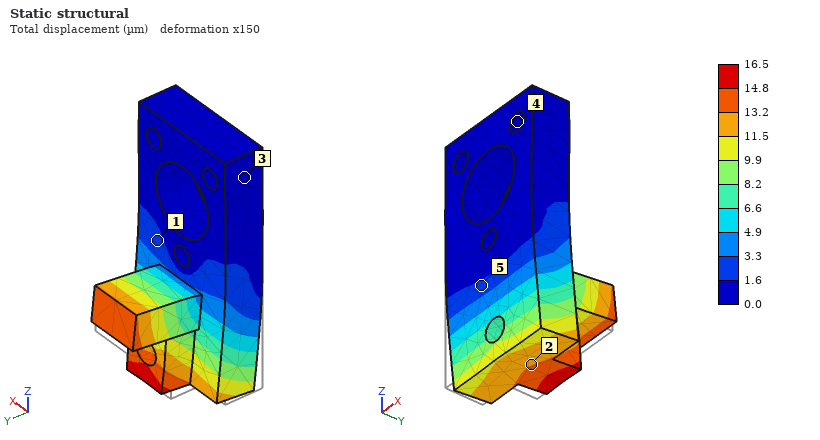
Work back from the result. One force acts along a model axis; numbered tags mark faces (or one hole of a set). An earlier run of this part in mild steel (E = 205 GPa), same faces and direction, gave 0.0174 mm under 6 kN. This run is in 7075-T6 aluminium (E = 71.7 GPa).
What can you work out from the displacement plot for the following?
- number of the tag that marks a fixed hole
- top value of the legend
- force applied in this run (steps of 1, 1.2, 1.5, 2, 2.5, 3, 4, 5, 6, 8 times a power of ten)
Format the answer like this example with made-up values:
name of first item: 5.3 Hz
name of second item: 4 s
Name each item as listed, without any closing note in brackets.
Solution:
number of the tag that marks a fixed hole: 4
top value of the legend: 16.5 µm
force applied in this run: 2 kN
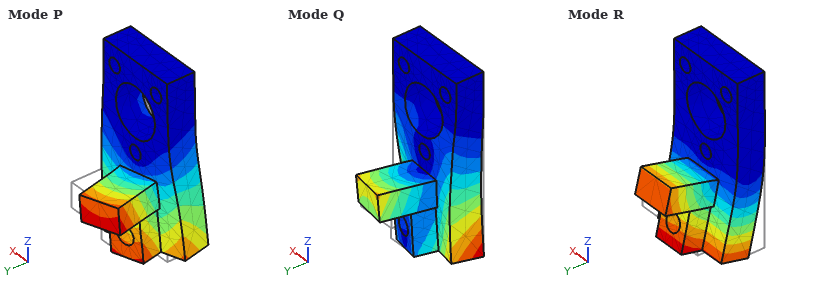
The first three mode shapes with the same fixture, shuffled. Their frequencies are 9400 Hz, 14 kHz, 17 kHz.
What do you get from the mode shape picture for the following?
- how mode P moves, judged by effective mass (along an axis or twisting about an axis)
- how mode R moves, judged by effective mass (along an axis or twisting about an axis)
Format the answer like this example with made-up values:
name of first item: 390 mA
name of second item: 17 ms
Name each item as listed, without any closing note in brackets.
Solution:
how mode P moves, judged by effective mass: along X
how mode R moves, judged by effective mass: along Y
